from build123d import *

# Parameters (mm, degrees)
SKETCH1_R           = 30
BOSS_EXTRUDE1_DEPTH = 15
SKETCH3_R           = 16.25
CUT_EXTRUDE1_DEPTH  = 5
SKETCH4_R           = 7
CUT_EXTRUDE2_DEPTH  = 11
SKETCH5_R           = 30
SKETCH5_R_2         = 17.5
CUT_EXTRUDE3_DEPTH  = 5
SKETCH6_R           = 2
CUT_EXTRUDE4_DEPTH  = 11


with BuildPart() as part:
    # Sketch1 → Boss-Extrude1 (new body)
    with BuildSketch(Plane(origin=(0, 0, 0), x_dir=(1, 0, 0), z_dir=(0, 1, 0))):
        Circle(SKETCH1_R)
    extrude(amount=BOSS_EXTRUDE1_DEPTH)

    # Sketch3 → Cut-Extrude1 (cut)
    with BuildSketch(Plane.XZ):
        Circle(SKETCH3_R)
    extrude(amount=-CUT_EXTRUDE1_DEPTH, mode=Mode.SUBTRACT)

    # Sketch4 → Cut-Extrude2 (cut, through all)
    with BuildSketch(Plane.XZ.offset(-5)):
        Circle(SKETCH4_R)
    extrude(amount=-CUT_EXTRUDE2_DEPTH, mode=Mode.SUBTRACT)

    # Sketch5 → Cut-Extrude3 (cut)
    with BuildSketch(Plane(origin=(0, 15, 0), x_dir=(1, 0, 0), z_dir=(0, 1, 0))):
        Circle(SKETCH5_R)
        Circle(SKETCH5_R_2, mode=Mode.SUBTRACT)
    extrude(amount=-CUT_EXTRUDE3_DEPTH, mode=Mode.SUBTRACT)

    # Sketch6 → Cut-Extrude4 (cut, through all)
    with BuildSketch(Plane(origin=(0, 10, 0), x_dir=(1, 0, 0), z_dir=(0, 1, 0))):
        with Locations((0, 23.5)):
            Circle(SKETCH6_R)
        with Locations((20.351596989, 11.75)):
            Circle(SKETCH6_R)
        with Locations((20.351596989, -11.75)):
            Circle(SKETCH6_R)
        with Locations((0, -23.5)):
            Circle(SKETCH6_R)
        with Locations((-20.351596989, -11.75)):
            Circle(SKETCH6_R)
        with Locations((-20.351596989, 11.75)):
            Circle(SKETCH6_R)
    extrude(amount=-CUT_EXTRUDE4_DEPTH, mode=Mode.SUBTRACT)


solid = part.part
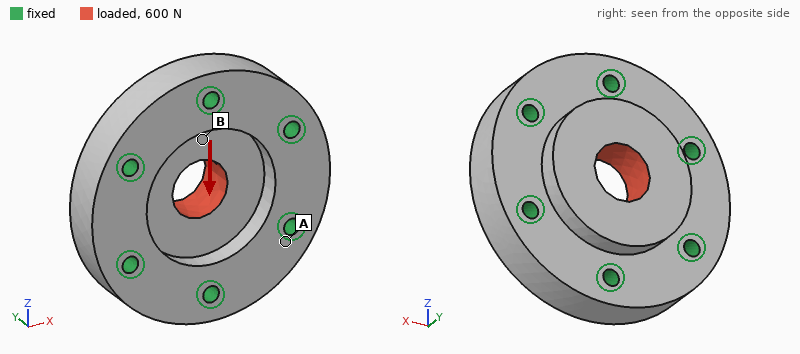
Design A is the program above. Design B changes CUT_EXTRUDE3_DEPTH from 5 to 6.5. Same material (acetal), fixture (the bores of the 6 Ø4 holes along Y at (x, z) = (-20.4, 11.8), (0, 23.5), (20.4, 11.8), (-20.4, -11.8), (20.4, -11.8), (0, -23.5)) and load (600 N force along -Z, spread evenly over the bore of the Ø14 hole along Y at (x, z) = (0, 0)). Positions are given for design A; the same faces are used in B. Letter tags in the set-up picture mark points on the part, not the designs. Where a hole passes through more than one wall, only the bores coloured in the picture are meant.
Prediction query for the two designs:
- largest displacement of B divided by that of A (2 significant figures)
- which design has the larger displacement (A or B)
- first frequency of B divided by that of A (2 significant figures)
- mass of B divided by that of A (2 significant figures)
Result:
1.2
B
0.95
0.90
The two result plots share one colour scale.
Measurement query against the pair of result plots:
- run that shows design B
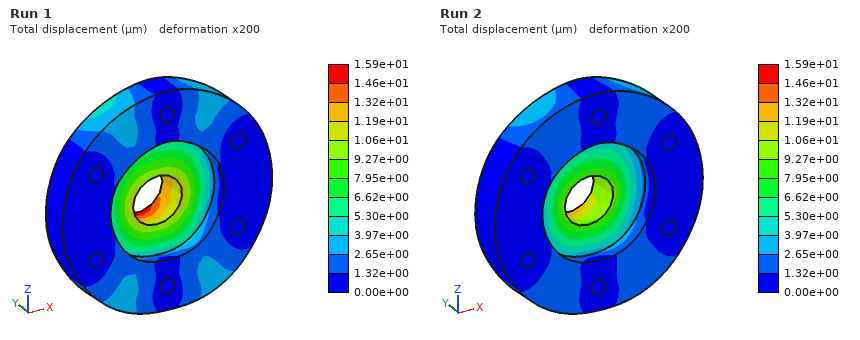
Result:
Run 1
